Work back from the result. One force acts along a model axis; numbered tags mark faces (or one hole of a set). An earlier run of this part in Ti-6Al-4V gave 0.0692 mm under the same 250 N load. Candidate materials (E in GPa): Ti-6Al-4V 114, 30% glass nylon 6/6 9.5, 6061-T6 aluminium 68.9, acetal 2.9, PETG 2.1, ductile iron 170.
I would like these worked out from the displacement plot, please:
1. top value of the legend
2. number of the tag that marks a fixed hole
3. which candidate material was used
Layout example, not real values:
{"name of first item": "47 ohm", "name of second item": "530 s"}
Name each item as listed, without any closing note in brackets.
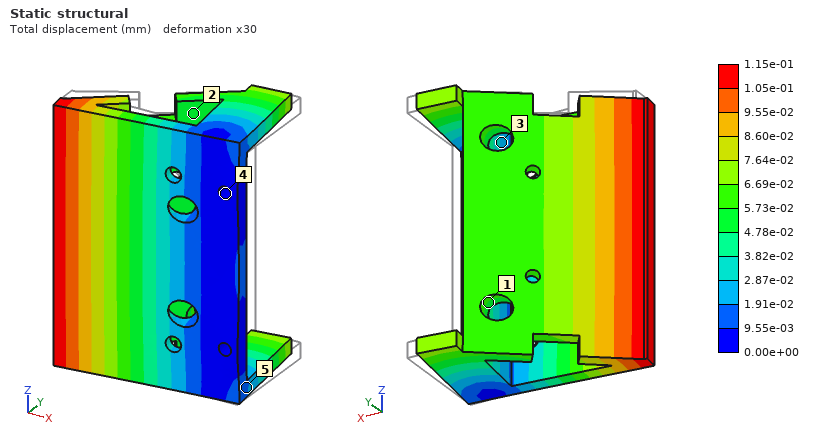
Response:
{"top value of the legend": "1.15e-01 mm", "number of the tag that marks a fixed hole": "4", "which candidate material was used": "6061-T6 aluminium"}
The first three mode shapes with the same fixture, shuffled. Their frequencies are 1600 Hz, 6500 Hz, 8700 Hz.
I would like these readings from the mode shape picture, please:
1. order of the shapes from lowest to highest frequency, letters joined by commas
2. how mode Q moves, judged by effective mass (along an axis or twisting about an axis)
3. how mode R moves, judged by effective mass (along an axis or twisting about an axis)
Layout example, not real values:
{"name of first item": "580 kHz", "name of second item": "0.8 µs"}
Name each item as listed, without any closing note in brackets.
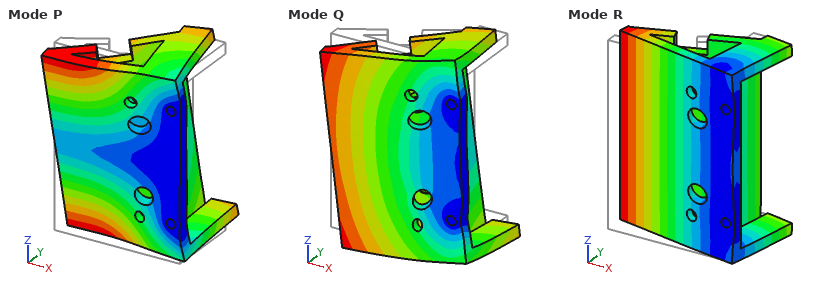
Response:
{"order of the shapes from lowest to highest frequency, letters joined by commas": "R, P, Q", "how mode Q moves, judged by effective mass": "along Z", "how mode R moves, judged by effective mass": "along Y"}
